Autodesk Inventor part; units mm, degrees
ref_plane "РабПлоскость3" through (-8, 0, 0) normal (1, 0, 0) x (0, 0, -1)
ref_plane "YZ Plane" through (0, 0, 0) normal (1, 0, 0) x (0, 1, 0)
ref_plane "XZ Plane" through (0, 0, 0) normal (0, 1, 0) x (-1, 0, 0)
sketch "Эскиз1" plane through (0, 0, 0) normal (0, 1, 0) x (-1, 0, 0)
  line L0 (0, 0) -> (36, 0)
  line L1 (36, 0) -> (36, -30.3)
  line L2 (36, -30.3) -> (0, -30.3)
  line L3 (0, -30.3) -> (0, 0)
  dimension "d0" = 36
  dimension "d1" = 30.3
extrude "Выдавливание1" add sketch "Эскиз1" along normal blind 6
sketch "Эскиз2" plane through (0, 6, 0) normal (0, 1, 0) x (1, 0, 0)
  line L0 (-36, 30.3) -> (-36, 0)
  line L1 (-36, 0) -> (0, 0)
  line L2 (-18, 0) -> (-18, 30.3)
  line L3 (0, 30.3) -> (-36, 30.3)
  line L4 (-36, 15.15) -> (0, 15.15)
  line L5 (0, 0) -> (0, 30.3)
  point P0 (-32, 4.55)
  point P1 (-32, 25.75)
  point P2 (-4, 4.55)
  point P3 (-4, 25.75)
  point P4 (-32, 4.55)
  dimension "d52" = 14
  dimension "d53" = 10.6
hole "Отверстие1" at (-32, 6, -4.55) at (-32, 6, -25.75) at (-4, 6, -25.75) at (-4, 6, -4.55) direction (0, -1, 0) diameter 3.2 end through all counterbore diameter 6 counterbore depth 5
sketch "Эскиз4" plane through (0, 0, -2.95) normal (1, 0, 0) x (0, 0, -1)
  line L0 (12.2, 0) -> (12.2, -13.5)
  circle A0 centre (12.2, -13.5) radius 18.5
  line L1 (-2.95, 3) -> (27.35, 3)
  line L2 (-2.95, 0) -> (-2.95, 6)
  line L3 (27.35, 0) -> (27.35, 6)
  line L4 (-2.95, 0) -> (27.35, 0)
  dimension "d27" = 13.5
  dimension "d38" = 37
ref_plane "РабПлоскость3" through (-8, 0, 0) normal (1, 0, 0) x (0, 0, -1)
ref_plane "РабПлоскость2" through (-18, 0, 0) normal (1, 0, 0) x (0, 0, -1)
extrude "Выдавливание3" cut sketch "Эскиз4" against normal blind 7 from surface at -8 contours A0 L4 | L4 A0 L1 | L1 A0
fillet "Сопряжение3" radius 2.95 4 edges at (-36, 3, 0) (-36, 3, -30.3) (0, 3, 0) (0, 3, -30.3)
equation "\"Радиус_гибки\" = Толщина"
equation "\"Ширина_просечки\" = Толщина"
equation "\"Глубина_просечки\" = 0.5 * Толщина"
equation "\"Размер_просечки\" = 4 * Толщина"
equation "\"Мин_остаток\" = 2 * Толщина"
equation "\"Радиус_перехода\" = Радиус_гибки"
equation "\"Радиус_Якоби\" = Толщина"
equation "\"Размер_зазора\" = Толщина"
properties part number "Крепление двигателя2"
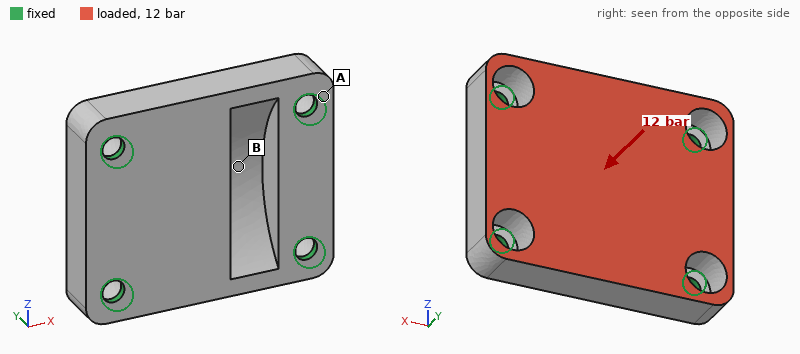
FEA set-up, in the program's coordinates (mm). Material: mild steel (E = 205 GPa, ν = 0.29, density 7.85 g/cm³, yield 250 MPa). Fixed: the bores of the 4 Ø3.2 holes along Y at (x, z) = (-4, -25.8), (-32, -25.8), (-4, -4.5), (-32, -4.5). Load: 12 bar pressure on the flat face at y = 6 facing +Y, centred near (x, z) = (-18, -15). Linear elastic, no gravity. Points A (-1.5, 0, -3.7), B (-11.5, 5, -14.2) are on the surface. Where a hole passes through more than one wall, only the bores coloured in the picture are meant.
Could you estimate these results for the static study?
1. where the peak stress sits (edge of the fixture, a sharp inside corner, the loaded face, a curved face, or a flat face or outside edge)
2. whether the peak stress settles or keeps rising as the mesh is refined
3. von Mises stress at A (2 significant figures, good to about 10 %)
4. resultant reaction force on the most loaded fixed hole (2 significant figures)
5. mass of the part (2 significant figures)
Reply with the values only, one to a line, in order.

edge of the fixture
keeps rising
25 MPa
370 N
42 g
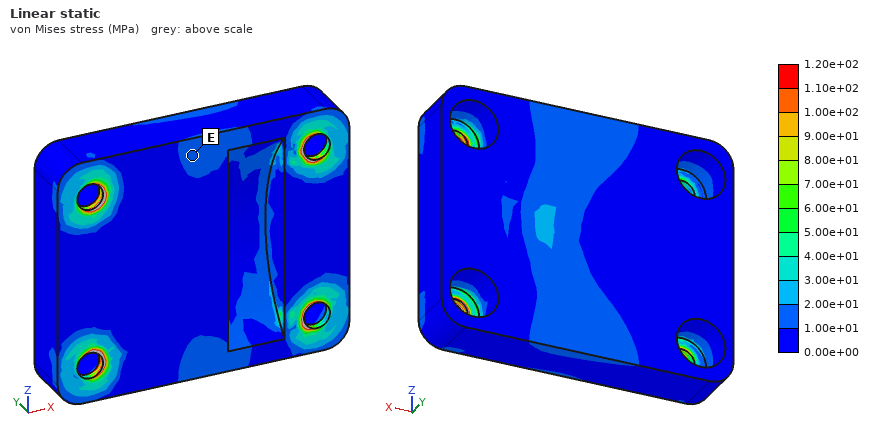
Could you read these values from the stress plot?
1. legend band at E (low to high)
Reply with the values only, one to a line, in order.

1.00e+01 to 2.00e+01 MPa
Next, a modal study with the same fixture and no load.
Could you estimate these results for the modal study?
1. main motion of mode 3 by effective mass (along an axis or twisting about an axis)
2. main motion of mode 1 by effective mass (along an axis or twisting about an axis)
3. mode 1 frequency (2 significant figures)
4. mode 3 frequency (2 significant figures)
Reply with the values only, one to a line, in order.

along X
along Y
17 kHz
27 kHz
